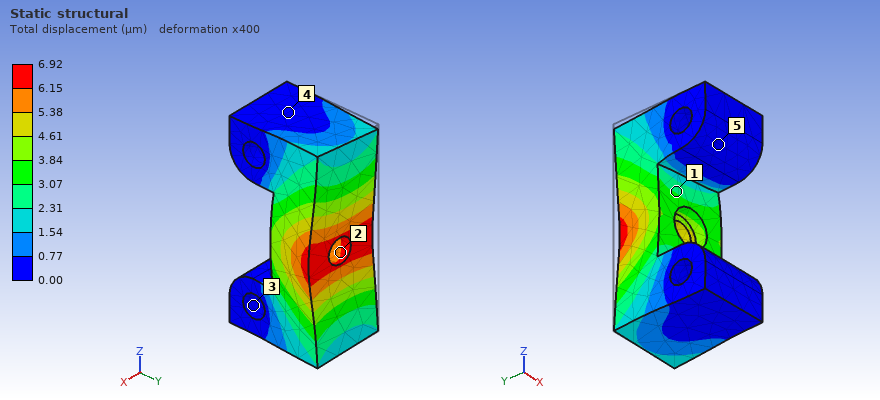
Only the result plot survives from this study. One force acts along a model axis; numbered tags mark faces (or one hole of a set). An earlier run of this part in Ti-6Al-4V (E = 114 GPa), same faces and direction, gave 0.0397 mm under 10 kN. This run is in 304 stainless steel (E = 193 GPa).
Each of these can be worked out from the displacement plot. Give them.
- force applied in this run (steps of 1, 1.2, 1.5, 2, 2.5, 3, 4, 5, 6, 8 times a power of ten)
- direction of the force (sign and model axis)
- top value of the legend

3 kN
+X
6.92 µm
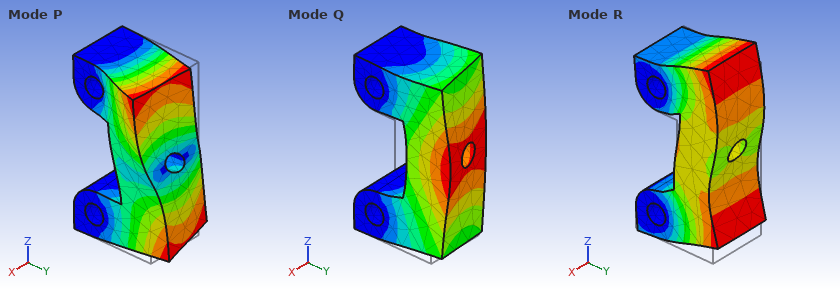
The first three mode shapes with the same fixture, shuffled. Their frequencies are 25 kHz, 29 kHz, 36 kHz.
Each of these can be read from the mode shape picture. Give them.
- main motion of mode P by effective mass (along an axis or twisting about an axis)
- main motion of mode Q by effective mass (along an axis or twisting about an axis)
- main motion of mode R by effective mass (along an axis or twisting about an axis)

twisting about Y
along X
along Z
